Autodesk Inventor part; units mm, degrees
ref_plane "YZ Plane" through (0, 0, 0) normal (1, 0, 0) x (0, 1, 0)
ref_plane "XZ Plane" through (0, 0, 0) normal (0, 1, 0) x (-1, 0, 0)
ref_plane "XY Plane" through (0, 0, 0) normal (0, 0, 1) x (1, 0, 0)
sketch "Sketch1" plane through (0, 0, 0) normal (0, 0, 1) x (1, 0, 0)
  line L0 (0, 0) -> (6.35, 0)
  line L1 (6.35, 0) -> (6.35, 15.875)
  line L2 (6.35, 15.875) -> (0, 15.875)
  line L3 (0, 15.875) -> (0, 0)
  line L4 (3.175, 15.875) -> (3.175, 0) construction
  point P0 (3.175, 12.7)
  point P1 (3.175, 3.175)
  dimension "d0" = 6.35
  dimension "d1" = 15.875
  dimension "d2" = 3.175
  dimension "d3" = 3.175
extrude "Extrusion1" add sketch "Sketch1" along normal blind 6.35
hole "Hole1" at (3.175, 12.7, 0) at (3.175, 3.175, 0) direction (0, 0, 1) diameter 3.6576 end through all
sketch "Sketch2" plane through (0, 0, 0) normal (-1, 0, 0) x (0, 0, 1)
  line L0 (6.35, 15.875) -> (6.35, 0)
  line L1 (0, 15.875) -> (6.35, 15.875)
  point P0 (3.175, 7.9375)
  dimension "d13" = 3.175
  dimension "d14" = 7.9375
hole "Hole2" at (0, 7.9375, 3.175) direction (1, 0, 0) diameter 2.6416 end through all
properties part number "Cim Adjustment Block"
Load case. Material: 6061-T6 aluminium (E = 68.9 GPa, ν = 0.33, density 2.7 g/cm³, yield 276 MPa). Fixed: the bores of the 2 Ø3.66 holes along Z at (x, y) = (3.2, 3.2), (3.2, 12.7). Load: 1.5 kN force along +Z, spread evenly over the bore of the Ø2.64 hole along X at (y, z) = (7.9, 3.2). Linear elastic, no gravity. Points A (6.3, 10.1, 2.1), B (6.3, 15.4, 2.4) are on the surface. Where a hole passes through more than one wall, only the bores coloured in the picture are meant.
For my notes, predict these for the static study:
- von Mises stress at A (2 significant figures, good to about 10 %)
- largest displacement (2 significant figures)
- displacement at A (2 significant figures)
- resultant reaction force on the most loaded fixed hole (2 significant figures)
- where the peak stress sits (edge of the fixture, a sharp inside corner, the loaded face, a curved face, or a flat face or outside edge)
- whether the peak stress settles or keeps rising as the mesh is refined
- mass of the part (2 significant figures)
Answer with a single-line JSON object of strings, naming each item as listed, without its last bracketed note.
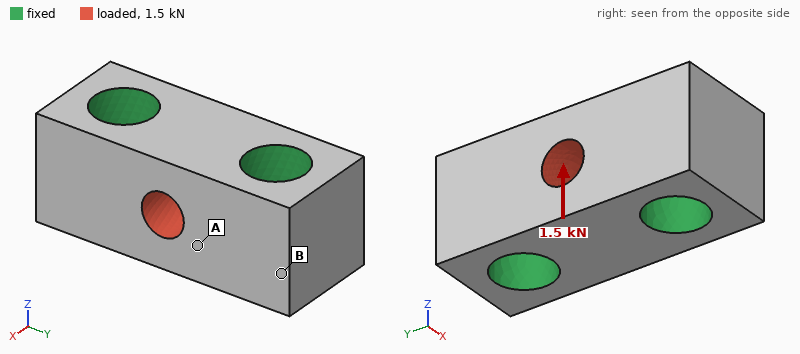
{"von Mises stress at A": "32 MPa", "largest displacement": "3.1 µm", "displacement at A": "1.3 µm", "resultant reaction force on the most loaded fixed hole": "750 N", "where the peak stress sits": "edge of the fixture", "whether the peak stress settles or keeps rising as the mesh is refined": "keeps rising", "mass of the part": "1.3 g"}
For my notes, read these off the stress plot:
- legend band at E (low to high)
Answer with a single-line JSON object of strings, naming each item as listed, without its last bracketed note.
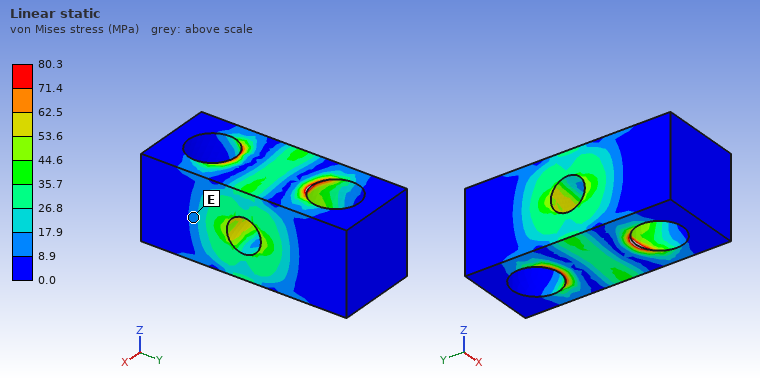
{"legend band at E": "8.9 to 17.9 MPa"}
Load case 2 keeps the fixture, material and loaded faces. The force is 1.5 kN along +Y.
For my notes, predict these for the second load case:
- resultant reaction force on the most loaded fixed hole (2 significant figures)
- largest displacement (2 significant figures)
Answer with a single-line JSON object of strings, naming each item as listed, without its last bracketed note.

{"resultant reaction force on the most loaded fixed hole": "750 N", "largest displacement": "1.3 µm"}
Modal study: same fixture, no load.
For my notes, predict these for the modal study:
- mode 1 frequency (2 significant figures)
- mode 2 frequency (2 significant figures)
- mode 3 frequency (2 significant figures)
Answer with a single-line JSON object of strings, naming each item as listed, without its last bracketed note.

{"mode 1 frequency": "210 kHz", "mode 2 frequency": "210 kHz", "mode 3 frequency": "220 kHz"}
